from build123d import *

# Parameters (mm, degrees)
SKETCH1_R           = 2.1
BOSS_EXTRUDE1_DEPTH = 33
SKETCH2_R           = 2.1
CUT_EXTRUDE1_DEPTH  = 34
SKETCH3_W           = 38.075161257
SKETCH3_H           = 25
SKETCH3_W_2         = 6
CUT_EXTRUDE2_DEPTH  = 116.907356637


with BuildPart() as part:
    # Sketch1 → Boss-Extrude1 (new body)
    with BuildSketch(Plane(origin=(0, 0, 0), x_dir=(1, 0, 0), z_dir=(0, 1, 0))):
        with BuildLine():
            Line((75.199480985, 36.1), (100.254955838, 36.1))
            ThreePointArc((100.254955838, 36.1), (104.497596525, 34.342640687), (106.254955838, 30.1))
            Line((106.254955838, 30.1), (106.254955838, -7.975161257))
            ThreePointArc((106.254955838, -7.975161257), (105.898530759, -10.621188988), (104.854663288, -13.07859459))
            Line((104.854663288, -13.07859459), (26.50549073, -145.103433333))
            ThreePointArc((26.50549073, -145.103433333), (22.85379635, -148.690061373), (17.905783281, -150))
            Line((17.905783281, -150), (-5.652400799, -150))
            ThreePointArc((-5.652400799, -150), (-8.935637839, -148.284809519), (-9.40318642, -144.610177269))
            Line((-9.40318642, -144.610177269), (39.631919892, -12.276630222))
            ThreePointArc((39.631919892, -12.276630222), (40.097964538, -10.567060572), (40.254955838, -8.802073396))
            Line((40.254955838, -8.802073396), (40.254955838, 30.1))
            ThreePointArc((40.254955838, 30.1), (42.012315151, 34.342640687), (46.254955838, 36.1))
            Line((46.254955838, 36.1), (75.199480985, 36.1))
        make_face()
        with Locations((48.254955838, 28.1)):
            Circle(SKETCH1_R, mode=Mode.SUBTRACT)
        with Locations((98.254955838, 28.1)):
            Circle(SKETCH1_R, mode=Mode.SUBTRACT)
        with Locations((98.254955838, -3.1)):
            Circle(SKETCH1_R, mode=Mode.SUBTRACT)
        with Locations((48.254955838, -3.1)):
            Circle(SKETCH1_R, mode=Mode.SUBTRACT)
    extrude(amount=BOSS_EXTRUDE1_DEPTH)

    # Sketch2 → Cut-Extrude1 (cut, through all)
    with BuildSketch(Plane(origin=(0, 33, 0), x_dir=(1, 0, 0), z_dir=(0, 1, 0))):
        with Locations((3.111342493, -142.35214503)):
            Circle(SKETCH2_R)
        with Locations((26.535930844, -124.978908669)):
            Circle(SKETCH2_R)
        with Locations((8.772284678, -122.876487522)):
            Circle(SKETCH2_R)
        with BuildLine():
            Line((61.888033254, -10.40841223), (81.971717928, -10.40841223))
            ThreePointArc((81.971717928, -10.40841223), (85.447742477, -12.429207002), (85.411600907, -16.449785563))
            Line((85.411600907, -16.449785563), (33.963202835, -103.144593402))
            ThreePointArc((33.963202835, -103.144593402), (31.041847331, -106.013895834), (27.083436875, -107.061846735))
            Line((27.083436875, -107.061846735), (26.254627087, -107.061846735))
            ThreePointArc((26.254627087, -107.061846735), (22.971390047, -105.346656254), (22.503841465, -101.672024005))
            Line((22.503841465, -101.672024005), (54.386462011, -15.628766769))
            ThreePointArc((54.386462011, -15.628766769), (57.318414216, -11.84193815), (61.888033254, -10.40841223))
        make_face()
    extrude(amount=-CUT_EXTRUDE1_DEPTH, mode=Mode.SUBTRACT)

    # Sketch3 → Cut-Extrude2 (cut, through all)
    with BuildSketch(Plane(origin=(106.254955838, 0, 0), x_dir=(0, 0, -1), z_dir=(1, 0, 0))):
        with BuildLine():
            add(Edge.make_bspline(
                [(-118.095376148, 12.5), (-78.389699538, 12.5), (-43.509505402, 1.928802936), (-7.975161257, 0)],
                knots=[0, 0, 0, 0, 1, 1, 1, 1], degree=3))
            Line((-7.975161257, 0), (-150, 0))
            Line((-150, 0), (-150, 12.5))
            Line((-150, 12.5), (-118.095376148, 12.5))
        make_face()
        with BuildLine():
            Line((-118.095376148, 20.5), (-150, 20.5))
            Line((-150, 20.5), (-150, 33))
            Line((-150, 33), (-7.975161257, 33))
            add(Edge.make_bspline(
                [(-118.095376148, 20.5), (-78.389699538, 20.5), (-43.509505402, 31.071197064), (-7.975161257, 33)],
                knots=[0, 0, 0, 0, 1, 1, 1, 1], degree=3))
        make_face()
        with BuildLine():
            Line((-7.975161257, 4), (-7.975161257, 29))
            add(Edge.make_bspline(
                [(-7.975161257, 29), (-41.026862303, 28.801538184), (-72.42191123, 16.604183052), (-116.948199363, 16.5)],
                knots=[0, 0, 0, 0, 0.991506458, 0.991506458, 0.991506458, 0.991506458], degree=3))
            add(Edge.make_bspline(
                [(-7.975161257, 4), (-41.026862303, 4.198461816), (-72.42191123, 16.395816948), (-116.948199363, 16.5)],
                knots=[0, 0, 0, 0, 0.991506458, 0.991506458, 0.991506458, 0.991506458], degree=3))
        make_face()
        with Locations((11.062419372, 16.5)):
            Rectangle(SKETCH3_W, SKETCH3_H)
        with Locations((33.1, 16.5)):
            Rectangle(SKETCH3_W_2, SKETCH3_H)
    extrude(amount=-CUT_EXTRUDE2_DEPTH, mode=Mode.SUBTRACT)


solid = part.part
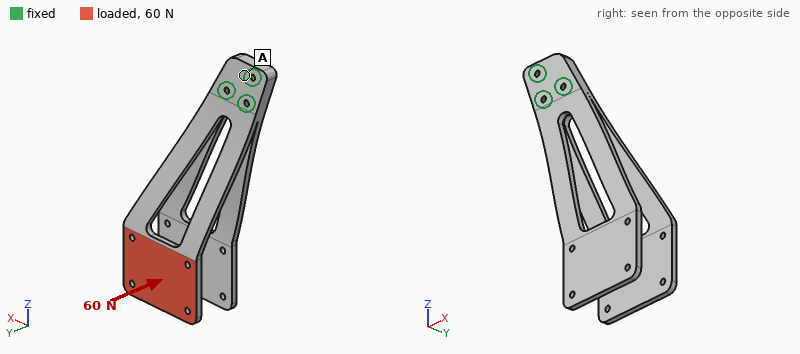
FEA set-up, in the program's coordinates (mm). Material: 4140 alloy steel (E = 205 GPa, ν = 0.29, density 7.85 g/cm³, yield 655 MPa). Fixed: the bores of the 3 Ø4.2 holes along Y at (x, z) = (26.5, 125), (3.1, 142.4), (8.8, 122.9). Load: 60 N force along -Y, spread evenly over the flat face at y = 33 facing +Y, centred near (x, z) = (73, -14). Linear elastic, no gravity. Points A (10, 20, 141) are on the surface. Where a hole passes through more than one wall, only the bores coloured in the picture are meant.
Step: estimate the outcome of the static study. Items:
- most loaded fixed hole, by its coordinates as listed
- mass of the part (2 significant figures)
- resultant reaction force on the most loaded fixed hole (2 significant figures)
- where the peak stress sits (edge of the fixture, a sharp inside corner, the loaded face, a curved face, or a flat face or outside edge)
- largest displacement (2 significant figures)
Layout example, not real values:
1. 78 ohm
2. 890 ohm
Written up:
1. (26.5, 125)
2. 490 g
3. 140 N
4. a curved face
5. 2.3 mm
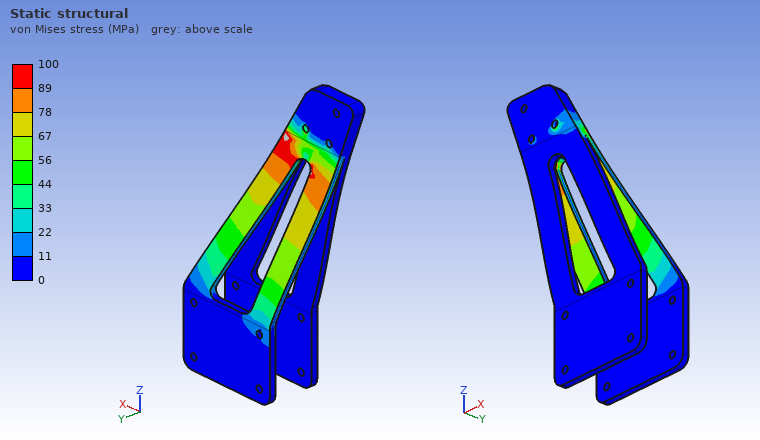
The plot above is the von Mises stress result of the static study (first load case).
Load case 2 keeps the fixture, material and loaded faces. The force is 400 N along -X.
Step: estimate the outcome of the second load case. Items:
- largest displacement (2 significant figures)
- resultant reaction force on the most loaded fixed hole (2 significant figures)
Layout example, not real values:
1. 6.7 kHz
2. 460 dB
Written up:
1. 0.33 mm
2. 2.2 kN
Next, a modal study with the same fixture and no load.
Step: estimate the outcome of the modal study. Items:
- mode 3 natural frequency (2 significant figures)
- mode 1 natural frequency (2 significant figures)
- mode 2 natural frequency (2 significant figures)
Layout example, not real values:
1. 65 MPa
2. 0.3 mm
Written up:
1. 420 Hz
2. 90 Hz
3. 91 Hz
